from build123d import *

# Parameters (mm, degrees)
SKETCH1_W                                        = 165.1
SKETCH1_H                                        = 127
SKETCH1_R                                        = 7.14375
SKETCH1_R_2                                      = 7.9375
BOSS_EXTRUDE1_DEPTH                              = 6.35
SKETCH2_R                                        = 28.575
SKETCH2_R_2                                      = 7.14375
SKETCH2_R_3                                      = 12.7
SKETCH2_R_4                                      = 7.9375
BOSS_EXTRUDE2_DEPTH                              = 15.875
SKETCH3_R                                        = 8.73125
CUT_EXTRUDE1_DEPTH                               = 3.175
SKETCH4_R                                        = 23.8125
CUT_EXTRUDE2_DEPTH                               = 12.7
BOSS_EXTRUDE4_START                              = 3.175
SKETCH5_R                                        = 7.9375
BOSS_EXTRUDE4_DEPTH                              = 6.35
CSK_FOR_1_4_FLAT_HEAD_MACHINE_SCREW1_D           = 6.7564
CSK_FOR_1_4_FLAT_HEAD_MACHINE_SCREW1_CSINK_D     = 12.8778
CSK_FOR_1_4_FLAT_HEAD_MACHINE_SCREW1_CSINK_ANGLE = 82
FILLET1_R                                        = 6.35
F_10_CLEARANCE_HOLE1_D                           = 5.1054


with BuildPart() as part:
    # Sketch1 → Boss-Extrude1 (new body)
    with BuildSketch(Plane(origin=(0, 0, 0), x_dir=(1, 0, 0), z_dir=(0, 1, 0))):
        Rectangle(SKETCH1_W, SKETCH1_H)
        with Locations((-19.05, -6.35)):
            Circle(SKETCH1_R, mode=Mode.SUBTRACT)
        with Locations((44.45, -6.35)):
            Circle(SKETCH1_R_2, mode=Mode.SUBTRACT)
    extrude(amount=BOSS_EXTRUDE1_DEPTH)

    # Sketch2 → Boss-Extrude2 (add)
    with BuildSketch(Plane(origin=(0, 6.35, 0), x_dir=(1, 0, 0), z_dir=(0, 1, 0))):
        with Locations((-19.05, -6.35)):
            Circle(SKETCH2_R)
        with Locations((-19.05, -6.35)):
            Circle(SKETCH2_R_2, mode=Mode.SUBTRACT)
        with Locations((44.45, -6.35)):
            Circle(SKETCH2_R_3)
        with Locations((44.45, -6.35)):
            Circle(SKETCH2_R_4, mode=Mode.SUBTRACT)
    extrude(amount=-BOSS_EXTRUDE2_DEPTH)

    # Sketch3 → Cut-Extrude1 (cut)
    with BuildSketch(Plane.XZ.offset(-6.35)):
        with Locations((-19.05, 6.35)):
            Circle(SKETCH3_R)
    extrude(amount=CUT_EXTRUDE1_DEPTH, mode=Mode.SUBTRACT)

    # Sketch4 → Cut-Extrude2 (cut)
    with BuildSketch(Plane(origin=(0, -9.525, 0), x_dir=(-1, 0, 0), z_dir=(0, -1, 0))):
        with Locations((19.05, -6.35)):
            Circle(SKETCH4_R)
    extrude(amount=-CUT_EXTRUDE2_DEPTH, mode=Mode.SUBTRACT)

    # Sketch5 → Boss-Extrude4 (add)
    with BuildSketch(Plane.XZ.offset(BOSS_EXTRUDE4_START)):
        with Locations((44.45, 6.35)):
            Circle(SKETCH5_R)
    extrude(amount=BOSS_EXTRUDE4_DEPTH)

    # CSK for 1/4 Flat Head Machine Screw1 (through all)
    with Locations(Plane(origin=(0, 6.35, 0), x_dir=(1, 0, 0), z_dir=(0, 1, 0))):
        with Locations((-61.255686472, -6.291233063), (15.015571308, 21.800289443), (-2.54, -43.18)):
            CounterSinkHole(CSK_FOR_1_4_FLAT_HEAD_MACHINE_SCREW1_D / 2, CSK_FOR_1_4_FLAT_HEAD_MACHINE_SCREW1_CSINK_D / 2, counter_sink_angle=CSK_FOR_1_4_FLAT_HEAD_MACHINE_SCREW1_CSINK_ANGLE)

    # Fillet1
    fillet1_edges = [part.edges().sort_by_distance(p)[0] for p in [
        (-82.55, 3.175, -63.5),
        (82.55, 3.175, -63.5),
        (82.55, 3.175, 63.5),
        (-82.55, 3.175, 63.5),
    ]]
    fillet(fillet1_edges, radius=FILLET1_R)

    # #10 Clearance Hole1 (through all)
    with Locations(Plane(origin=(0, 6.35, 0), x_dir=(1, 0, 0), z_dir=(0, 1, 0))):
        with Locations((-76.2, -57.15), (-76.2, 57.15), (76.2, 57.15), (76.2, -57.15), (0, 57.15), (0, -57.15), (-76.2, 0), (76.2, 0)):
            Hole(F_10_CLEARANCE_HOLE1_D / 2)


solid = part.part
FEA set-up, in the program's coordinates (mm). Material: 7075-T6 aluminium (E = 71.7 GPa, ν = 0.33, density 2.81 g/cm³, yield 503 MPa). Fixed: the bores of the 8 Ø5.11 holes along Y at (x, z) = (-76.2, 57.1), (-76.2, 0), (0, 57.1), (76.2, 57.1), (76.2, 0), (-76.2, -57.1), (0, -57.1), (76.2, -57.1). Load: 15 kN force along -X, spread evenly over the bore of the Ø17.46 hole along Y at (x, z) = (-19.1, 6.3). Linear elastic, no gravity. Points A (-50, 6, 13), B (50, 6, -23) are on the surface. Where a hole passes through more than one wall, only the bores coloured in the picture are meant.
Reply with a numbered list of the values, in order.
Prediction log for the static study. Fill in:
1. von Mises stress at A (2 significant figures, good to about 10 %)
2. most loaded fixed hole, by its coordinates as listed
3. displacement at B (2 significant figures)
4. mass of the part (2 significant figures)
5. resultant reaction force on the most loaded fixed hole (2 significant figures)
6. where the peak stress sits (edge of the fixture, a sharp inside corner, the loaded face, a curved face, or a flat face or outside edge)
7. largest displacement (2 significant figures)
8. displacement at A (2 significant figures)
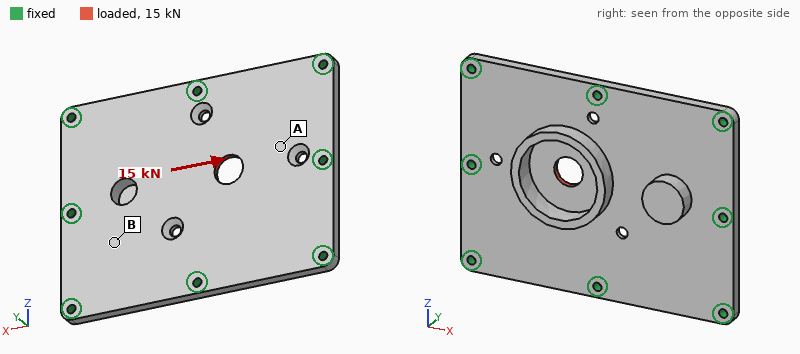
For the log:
1. 35 MPa
2. (-76.2, 0)
3. 7.9 µm
4. 380 g
5. 3.5 kN
6. the loaded face
7. 34 µm
8. 14 µm
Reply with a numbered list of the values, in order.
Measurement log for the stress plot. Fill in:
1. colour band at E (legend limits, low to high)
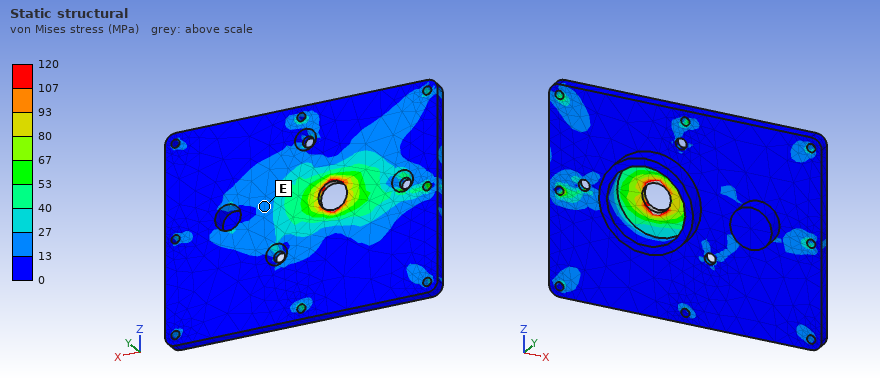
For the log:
1. 13 to 27 MPa
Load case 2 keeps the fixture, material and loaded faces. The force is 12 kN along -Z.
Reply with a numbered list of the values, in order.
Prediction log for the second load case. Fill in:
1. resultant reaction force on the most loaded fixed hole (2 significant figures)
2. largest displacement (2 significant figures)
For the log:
1. 3.3 kN
2. 30 µm
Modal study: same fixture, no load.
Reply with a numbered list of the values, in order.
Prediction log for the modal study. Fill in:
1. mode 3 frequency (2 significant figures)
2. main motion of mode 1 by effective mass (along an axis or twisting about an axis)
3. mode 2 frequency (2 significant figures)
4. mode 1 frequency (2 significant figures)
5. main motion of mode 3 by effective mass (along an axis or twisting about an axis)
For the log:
1. 4800 Hz
2. along Y
3. 4000 Hz
4. 2700 Hz
5. twisting about X
